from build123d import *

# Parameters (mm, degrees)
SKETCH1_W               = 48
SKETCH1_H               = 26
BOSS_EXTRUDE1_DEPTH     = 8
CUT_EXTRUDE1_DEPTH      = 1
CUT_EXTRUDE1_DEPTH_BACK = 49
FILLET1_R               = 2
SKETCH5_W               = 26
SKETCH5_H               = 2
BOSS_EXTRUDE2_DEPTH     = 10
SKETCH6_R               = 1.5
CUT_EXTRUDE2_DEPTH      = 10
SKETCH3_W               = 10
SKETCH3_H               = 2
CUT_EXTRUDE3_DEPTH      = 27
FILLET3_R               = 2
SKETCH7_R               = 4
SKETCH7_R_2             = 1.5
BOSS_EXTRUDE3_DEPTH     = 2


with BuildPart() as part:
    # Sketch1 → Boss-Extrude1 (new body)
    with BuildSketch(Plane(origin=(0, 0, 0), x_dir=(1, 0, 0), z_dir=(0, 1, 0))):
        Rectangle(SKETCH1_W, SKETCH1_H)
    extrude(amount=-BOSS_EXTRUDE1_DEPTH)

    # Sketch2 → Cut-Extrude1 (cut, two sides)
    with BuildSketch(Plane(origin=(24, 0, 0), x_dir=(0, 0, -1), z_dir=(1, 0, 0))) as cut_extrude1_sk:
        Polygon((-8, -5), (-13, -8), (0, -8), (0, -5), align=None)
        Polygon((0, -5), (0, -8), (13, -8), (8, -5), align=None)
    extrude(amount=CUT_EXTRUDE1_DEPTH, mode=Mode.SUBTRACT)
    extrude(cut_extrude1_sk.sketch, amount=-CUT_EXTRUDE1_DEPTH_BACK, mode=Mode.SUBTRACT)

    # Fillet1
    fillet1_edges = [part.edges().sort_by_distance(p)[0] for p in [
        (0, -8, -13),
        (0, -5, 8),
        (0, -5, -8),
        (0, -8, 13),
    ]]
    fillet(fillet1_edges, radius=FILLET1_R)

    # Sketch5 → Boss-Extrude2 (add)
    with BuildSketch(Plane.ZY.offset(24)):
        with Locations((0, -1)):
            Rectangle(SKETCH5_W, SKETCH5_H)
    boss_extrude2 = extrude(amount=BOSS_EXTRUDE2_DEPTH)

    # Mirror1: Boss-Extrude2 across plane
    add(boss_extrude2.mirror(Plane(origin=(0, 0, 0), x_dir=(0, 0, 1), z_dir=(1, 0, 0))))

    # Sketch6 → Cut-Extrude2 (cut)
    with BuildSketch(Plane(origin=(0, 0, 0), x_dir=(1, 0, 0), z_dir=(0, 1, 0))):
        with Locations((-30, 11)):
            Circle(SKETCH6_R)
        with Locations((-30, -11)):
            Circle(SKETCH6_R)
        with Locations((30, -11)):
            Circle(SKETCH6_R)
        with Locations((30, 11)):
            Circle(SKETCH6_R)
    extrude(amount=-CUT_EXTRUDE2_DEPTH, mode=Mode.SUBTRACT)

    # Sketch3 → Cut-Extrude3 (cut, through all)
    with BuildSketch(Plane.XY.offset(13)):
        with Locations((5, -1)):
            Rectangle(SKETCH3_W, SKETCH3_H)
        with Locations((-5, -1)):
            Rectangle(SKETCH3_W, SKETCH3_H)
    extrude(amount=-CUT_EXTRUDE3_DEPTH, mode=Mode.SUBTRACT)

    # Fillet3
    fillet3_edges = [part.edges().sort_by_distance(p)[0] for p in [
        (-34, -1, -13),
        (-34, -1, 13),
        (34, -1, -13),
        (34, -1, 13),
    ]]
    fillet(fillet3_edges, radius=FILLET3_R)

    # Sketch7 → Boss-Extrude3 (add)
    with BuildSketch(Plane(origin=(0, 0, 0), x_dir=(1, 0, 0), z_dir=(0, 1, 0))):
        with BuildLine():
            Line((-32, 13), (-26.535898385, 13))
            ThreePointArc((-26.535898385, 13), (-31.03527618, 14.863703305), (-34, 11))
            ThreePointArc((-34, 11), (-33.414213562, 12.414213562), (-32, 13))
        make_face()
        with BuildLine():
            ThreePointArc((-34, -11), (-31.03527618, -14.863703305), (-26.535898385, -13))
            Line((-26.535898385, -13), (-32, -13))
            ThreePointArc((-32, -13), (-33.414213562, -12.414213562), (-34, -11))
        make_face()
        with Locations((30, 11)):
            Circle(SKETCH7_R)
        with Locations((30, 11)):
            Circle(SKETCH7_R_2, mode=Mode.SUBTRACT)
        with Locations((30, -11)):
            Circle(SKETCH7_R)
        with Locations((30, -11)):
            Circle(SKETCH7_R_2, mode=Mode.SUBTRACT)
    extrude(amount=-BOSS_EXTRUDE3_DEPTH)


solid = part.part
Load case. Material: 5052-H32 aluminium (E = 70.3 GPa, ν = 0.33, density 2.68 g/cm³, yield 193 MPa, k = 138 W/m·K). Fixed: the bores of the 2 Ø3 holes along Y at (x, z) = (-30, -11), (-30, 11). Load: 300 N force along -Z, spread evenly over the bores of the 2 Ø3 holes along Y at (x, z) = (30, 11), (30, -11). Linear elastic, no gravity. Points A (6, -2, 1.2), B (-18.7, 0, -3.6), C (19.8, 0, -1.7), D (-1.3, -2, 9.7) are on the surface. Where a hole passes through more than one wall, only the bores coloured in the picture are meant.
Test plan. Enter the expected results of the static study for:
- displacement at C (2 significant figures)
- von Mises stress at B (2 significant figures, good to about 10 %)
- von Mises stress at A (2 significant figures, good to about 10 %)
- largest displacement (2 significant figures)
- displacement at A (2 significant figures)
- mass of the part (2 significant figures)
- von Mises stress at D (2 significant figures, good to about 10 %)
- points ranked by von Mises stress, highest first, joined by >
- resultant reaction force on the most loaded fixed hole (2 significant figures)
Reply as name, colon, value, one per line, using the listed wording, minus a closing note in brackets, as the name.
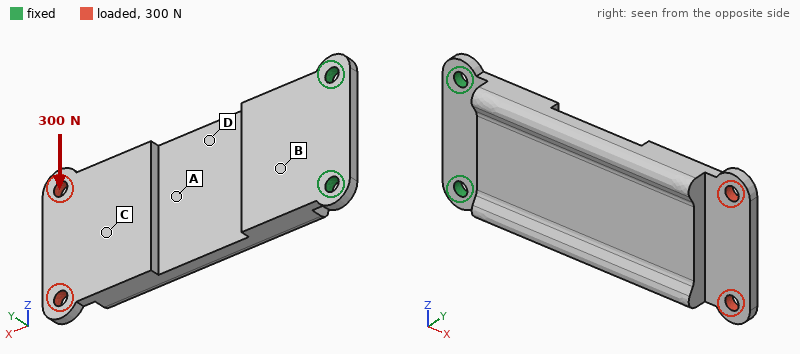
displacement at C: 0.080 mm
von Mises stress at B: 38 MPa
von Mises stress at A: 16 MPa
largest displacement: 0.12 mm
displacement at A: 0.046 mm
mass of the part: 18 g
von Mises stress at D: 28 MPa
points ranked by von Mises stress, highest first, joined by >: B > D > A > C
resultant reaction force on the most loaded fixed hole: 820 N
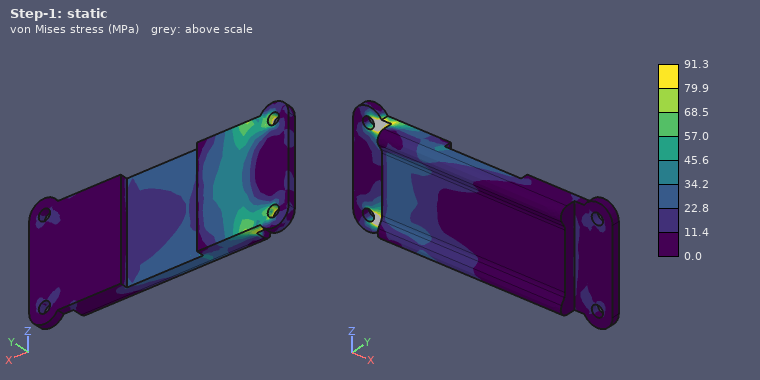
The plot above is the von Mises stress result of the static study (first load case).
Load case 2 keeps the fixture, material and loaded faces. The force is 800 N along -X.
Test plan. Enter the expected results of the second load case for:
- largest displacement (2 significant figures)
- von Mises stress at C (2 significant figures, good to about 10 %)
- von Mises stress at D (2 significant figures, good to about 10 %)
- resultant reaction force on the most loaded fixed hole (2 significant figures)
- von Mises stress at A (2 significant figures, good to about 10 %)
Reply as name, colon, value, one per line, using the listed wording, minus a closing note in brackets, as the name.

largest displacement: 0.29 mm
von Mises stress at C: 11 MPa
von Mises stress at D: 47 MPa
resultant reaction force on the most loaded fixed hole: 410 N
von Mises stress at A: 45 MPa
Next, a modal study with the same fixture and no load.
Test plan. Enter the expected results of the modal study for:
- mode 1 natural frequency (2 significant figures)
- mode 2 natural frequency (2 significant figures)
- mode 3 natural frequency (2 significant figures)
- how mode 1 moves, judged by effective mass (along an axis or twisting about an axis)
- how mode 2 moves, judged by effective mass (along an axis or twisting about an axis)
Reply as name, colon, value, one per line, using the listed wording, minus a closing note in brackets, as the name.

mode 1 natural frequency: 460 Hz
mode 2 natural frequency: 3400 Hz
mode 3 natural frequency: 4000 Hz
how mode 1 moves, judged by effective mass: along Y
how mode 2 moves, judged by effective mass: along Z
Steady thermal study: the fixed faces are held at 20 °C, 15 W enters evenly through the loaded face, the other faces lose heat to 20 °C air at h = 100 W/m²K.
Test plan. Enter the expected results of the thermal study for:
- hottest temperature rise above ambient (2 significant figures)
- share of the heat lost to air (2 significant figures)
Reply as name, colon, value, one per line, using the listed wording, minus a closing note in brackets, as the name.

hottest temperature rise above ambient: 56 K
share of the heat lost to air: 61 %
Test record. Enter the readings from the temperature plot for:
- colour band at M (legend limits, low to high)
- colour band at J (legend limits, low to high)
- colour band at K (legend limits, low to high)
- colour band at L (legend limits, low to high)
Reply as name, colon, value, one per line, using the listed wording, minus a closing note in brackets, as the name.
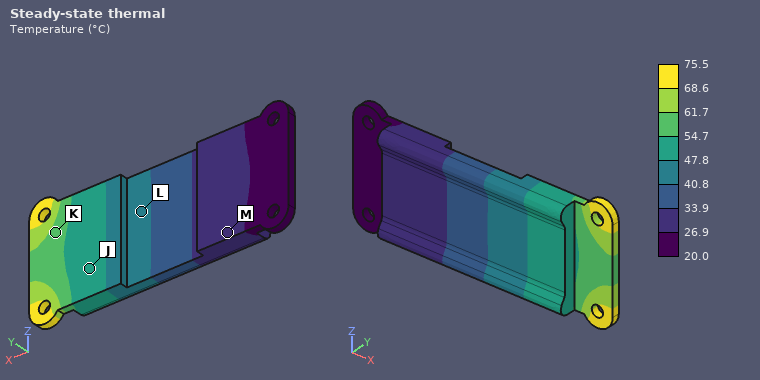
colour band at M: 26.9 to 33.9 °C
colour band at J: 47.8 to 54.7 °C
colour band at K: 54.7 to 61.7 °C
colour band at L: 40.8 to 47.8 °C
